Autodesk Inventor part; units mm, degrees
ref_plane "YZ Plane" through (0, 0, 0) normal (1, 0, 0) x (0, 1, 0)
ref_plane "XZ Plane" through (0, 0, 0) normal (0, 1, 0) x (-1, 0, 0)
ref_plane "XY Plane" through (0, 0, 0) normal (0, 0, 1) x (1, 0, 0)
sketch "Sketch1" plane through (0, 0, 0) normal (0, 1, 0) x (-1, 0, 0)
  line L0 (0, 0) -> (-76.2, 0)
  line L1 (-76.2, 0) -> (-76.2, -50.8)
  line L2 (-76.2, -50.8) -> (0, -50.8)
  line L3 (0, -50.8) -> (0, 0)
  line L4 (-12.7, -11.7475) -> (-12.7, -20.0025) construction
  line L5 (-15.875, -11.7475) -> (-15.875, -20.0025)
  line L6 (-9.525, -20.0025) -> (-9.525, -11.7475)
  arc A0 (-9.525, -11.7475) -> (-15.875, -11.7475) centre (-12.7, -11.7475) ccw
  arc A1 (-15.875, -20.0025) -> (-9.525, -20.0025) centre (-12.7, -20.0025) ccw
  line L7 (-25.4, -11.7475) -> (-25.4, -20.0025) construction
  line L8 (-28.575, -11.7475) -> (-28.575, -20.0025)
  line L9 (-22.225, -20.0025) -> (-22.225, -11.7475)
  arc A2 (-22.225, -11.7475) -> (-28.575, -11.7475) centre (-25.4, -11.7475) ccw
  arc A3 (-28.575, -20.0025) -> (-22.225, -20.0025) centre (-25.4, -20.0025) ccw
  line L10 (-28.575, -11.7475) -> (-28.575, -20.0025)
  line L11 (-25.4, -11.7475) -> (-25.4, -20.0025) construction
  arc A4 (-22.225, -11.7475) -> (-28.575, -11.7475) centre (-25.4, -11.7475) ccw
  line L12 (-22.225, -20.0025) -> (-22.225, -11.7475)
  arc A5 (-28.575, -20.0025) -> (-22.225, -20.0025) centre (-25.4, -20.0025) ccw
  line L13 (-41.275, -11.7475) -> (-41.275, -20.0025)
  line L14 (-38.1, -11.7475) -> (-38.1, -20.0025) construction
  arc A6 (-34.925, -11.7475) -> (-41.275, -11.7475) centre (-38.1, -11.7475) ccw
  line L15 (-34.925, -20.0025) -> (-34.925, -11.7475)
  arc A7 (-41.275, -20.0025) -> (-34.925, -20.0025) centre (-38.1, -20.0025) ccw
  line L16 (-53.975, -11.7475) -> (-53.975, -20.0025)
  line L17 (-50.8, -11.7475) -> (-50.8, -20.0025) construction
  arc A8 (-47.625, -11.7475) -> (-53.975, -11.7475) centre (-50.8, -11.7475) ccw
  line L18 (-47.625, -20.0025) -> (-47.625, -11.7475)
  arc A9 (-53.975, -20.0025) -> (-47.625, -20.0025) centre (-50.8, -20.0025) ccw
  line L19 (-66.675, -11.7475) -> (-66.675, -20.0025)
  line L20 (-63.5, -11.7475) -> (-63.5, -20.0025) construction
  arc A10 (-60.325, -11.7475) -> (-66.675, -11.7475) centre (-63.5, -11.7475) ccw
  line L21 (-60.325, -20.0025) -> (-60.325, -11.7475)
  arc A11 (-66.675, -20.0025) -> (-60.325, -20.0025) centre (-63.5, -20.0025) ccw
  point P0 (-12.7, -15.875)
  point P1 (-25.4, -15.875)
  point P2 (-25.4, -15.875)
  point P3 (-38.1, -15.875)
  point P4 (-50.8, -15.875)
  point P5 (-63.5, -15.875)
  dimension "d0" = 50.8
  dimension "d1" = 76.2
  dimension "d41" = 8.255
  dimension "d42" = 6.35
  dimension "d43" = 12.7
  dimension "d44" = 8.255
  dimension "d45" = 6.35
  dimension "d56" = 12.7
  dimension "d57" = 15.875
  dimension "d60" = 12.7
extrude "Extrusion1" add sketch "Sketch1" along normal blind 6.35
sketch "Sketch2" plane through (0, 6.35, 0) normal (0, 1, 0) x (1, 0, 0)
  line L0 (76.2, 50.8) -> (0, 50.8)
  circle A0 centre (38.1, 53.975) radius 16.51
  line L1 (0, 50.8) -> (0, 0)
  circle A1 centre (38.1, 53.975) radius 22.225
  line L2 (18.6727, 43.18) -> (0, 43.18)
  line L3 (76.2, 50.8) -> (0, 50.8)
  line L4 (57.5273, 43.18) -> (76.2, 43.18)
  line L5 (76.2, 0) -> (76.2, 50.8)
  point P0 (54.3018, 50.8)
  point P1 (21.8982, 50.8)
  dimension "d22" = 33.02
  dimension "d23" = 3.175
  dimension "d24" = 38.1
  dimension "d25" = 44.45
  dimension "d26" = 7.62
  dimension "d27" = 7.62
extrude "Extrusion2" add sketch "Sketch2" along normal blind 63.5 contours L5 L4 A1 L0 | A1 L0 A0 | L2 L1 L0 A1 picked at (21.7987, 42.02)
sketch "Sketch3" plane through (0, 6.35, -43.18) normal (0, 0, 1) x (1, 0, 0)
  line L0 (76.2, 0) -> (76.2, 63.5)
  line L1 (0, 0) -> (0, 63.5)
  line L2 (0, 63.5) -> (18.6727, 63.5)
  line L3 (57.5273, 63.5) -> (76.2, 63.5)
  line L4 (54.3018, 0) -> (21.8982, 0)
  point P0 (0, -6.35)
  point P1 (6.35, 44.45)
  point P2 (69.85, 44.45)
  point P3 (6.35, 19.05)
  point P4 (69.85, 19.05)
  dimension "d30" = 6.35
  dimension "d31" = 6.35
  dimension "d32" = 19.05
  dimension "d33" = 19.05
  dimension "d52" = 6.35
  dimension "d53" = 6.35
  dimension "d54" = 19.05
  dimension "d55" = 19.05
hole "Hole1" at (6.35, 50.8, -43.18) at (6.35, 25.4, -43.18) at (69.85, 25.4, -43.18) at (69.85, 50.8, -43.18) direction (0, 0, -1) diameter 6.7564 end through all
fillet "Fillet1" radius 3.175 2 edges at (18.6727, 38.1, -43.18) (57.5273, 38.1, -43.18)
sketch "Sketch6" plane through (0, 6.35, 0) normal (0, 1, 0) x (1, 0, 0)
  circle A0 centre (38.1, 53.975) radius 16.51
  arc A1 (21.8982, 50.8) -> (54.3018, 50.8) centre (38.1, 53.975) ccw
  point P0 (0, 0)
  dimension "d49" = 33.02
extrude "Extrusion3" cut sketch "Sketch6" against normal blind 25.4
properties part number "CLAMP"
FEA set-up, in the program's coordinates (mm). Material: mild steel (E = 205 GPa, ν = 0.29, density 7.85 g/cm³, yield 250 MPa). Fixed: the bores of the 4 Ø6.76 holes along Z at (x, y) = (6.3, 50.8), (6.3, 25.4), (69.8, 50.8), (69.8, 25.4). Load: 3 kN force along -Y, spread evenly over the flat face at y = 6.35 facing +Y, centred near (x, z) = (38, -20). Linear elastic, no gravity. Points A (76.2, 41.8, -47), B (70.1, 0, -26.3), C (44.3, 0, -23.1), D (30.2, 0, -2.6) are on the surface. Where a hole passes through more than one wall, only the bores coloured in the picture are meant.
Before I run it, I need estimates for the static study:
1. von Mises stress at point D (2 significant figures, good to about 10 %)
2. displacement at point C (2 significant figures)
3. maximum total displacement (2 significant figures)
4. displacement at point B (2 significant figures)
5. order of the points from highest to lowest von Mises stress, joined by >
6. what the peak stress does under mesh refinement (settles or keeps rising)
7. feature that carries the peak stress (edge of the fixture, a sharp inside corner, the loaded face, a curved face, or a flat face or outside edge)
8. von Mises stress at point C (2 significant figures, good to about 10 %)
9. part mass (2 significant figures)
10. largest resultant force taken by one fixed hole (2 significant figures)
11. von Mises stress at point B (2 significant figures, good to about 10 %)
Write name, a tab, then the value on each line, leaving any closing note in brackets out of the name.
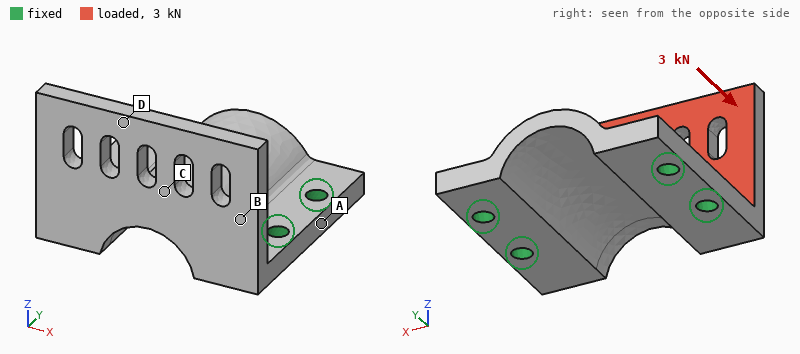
von Mises stress at point D	26 MPa
displacement at point C	0.050 mm
maximum total displacement	0.15 mm
displacement at point B	0.057 mm
order of the points from highest to lowest von Mises stress, joined by >	C > B > D > A
what the peak stress does under mesh refinement	keeps rising
feature that carries the peak stress	edge of the fixture
von Mises stress at point C	62 MPa
part mass	430 g
largest resultant force taken by one fixed hole	1.8 kN
von Mises stress at point B	46 MPa
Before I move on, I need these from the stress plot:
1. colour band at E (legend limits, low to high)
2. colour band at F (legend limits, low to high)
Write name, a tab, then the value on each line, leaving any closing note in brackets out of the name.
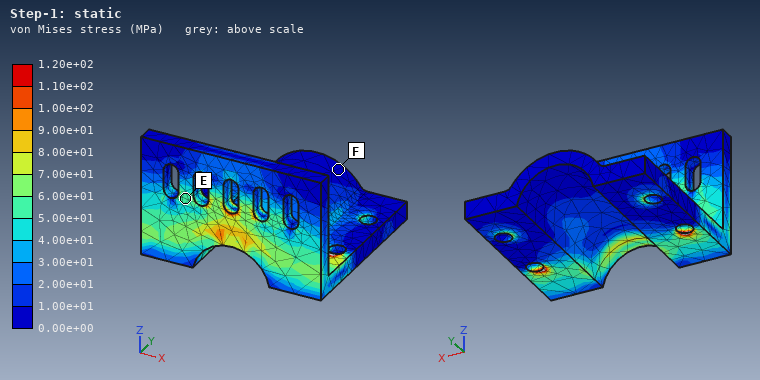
colour band at E	5.00e+01 to 6.00e+01 MPa
colour band at F	0.00e+00 to 1.00e+01 MPa
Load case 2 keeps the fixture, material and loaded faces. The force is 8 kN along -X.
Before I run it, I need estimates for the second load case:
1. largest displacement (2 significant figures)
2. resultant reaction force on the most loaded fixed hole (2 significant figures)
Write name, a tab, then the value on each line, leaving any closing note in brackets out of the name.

largest displacement	96 µm
resultant reaction force on the most loaded fixed hole	4.9 kN
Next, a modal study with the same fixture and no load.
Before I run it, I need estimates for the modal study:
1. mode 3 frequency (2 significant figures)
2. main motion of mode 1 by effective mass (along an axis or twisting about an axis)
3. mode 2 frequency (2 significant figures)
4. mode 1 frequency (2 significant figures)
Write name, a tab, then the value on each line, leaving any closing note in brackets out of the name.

mode 3 frequency	5500 Hz
main motion of mode 1 by effective mass	along Y
mode 2 frequency	3400 Hz
mode 1 frequency	2400 Hz
